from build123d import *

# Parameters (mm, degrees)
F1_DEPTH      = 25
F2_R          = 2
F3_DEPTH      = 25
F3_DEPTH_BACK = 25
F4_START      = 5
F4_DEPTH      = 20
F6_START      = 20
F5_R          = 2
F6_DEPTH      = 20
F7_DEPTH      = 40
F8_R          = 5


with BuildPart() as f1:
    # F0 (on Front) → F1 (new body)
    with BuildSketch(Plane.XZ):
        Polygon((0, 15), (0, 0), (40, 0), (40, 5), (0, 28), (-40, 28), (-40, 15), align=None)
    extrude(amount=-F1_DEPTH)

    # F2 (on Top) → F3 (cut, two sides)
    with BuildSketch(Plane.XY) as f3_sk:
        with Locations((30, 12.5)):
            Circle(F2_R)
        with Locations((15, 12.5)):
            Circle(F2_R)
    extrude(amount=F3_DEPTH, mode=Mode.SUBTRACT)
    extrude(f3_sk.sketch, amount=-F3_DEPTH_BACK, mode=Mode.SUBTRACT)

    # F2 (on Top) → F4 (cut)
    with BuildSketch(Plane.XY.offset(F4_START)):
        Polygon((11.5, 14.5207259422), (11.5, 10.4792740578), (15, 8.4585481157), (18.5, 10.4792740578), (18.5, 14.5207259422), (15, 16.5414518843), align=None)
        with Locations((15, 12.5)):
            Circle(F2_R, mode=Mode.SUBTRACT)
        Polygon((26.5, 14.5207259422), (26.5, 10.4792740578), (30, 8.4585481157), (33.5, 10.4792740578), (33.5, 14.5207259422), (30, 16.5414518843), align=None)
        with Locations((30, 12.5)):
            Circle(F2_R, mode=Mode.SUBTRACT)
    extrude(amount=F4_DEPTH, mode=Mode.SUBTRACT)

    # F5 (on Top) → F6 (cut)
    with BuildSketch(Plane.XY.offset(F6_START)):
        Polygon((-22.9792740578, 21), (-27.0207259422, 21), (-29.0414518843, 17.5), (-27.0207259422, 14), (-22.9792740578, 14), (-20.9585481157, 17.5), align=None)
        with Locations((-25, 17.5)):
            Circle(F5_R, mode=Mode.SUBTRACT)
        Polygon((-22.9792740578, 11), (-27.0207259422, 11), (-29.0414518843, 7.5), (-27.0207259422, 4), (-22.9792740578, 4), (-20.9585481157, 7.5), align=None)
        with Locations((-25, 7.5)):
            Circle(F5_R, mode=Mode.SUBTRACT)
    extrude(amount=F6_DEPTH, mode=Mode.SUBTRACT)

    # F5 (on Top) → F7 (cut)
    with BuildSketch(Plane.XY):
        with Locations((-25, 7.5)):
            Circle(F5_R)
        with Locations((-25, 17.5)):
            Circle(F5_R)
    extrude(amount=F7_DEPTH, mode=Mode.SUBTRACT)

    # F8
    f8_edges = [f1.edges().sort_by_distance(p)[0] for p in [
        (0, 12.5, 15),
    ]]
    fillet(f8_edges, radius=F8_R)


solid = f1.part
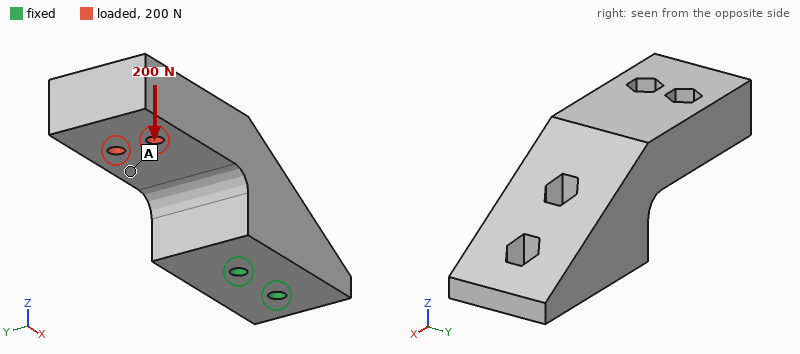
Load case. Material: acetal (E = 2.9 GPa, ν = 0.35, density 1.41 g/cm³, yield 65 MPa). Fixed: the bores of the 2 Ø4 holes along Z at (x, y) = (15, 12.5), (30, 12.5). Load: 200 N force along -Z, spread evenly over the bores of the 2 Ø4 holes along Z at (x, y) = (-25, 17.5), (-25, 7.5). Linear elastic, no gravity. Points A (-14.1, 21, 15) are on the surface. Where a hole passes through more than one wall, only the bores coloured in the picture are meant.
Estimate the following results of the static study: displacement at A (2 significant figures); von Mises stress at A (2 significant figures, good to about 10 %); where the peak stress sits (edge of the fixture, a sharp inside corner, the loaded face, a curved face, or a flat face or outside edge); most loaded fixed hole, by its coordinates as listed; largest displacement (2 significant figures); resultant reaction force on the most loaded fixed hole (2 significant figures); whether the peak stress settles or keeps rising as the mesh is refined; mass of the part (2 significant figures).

0.32 mm
3.1 MPa
edge of the fixture
(15, 12.5)
0.74 mm
640 N
keeps rising
39 g
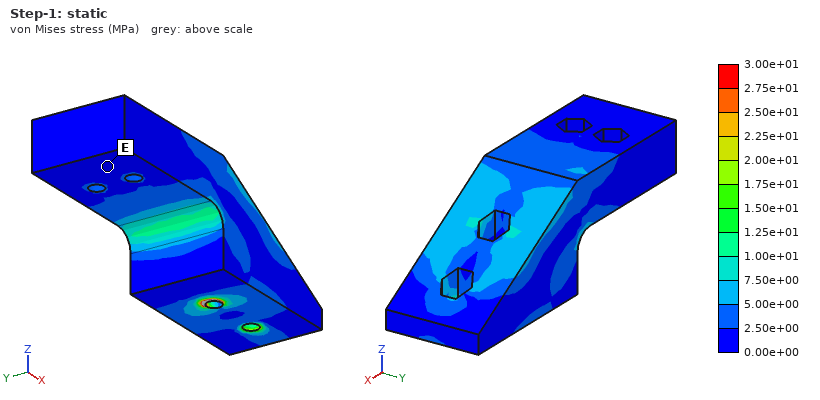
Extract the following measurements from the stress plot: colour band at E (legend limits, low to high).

0.00e+00 to 2.50e+00 MPa
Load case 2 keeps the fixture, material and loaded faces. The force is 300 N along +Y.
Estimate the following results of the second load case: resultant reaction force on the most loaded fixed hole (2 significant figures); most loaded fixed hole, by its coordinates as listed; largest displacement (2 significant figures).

940 N
(15, 12.5)
0.84 mm
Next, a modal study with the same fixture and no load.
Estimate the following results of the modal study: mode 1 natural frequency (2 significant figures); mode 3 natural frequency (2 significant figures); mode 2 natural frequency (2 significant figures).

790 Hz
1900 Hz
810 Hz
